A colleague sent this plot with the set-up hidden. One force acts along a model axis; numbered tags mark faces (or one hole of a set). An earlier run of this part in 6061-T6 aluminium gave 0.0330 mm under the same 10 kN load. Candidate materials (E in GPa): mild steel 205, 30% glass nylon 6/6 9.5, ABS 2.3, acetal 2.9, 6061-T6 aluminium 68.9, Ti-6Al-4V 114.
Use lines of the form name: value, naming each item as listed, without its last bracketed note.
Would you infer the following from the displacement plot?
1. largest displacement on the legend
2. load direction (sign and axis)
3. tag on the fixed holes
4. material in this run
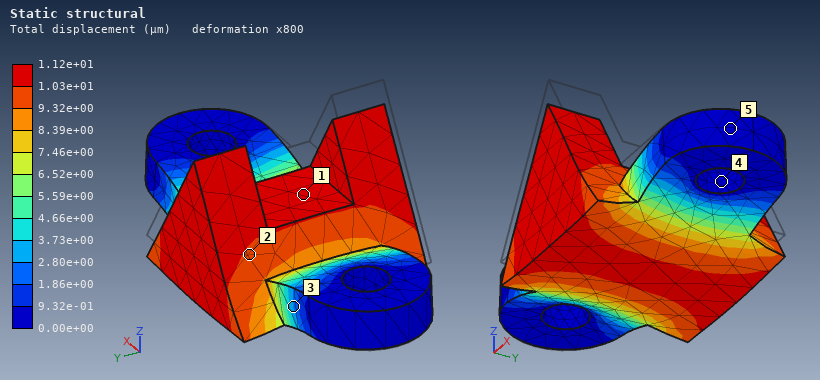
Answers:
largest displacement on the legend: 1.12e+01 µm
load direction: -Z
tag on the fixed holes: 4
material in this run: mild steel
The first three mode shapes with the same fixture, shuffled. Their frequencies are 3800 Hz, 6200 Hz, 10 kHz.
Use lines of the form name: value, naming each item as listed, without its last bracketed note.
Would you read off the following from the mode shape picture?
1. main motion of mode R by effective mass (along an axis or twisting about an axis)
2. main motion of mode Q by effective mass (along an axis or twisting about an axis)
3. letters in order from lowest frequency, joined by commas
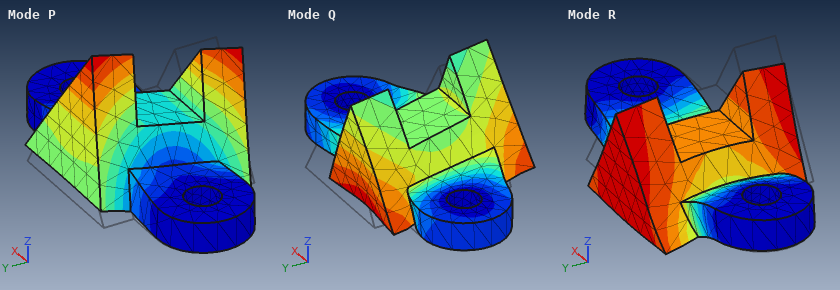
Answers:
main motion of mode R by effective mass: along Z
main motion of mode Q by effective mass: along Y
letters in order from lowest frequency, joined by commas: P, R, Q
